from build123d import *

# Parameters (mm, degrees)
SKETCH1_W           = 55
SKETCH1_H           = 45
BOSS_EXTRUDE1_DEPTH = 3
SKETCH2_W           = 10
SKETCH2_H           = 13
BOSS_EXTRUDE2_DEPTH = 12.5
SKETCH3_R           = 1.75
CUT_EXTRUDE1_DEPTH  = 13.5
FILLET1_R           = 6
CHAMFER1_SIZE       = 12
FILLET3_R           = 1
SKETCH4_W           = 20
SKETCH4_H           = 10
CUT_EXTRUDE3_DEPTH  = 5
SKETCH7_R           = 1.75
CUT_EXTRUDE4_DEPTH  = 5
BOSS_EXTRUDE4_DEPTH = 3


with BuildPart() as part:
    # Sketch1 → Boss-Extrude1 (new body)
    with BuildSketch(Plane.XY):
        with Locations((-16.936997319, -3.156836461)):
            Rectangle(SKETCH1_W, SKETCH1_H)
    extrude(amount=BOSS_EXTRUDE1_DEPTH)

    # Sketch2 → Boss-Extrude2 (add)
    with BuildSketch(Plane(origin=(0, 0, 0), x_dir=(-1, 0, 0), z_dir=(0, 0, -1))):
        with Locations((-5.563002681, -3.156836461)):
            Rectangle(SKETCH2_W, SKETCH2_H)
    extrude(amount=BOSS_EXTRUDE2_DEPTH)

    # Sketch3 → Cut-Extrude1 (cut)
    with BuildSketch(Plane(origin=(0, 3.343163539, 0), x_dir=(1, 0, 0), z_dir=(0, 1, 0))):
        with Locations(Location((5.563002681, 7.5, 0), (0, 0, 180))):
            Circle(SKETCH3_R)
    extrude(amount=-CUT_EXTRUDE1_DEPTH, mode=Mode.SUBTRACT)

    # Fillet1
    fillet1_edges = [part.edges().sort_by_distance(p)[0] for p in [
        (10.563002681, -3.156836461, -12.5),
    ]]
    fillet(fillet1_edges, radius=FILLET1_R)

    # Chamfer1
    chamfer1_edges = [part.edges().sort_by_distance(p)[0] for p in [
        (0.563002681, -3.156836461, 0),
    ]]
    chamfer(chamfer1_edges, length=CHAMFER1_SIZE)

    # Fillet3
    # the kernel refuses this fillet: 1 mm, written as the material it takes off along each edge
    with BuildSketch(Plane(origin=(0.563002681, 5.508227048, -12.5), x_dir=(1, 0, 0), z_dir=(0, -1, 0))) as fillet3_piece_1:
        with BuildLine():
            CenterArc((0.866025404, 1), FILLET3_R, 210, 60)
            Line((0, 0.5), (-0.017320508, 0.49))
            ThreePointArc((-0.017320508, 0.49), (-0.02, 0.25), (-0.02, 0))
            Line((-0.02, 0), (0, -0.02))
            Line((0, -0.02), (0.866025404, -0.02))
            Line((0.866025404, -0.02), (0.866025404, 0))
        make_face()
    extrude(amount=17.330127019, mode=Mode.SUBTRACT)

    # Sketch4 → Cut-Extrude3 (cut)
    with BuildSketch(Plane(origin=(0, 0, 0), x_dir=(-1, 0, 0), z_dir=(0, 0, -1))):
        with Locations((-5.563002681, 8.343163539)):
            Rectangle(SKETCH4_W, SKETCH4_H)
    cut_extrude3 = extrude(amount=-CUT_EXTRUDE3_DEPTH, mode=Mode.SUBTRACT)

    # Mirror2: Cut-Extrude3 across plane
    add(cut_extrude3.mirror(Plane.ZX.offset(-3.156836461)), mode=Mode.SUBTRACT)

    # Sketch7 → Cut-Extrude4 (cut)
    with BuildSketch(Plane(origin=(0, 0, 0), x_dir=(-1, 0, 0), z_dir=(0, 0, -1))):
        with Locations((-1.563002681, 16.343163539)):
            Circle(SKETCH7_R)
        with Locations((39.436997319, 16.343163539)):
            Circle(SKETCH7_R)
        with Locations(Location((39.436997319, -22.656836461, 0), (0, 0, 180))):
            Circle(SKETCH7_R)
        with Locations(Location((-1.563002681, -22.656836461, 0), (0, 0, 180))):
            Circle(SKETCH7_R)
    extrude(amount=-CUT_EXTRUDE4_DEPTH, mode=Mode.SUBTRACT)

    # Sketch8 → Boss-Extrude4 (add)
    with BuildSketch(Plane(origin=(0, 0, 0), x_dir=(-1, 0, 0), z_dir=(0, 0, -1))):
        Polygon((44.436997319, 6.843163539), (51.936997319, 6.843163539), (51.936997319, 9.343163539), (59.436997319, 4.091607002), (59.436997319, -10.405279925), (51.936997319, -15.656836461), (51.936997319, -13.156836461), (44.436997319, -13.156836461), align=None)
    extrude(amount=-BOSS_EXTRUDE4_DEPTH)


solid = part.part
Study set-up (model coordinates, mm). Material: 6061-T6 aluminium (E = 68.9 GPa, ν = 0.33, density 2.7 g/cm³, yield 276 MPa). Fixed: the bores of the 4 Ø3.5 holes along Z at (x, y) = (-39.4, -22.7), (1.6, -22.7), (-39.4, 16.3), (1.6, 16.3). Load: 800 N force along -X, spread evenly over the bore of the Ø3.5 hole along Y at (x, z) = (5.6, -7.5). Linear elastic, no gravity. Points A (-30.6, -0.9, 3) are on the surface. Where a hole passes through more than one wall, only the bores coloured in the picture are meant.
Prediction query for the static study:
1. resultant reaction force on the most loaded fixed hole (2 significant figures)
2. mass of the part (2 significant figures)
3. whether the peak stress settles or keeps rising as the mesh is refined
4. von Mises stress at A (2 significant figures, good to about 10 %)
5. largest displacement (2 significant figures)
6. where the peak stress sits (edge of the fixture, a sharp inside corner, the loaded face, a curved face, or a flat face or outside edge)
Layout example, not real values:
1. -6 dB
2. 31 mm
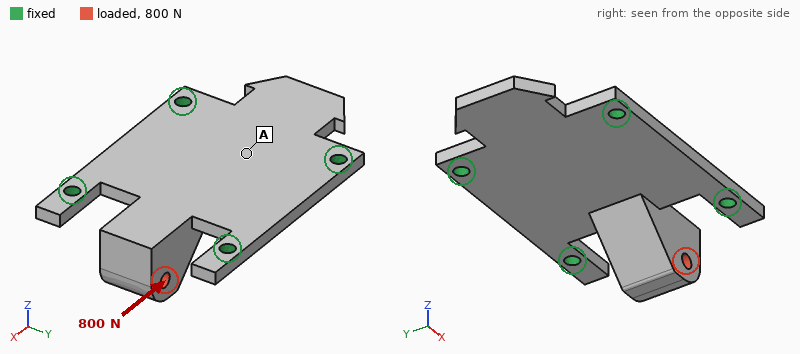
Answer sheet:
1. 320 N
2. 26 g
3. keeps rising
4. 14 MPa
5. 0.29 mm
6. a sharp inside corner
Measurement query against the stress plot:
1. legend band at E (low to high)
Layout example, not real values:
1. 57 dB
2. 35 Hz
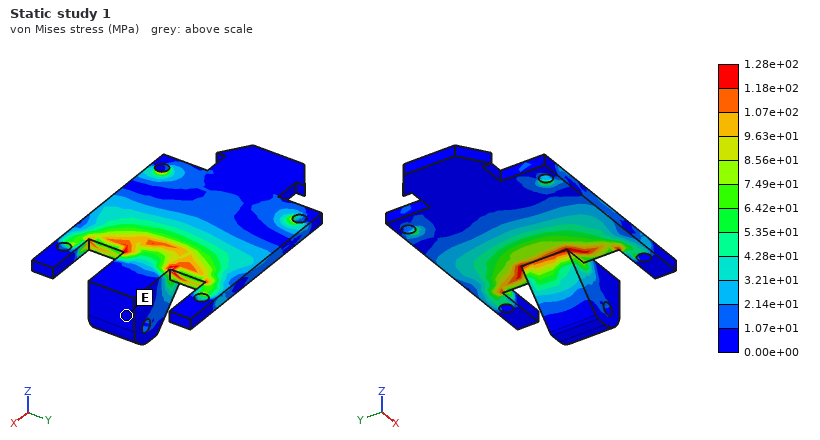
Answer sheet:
1. 0.00e+00 to 1.07e+01 MPa
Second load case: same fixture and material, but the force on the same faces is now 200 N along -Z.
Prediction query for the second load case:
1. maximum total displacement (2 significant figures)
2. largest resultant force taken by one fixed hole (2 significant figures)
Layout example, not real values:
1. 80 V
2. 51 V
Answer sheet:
1. 0.16 mm
2. 130 N
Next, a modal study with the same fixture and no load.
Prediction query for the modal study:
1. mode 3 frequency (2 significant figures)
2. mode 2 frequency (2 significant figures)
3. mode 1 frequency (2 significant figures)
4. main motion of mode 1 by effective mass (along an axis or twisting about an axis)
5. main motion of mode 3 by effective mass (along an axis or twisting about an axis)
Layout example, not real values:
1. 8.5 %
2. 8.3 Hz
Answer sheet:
1. 5700 Hz
2. 4300 Hz
3. 2400 Hz
4. along Z
5. along Z
